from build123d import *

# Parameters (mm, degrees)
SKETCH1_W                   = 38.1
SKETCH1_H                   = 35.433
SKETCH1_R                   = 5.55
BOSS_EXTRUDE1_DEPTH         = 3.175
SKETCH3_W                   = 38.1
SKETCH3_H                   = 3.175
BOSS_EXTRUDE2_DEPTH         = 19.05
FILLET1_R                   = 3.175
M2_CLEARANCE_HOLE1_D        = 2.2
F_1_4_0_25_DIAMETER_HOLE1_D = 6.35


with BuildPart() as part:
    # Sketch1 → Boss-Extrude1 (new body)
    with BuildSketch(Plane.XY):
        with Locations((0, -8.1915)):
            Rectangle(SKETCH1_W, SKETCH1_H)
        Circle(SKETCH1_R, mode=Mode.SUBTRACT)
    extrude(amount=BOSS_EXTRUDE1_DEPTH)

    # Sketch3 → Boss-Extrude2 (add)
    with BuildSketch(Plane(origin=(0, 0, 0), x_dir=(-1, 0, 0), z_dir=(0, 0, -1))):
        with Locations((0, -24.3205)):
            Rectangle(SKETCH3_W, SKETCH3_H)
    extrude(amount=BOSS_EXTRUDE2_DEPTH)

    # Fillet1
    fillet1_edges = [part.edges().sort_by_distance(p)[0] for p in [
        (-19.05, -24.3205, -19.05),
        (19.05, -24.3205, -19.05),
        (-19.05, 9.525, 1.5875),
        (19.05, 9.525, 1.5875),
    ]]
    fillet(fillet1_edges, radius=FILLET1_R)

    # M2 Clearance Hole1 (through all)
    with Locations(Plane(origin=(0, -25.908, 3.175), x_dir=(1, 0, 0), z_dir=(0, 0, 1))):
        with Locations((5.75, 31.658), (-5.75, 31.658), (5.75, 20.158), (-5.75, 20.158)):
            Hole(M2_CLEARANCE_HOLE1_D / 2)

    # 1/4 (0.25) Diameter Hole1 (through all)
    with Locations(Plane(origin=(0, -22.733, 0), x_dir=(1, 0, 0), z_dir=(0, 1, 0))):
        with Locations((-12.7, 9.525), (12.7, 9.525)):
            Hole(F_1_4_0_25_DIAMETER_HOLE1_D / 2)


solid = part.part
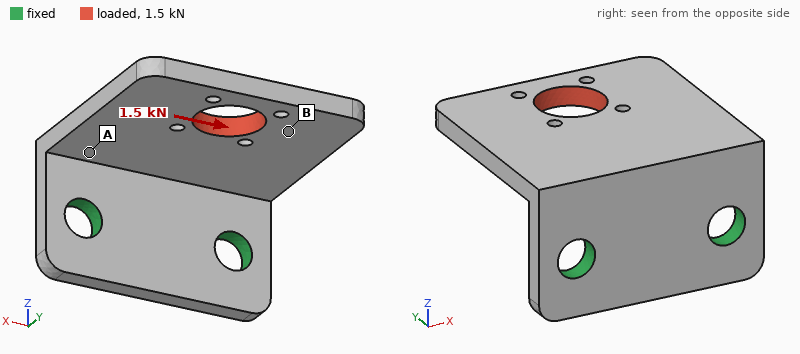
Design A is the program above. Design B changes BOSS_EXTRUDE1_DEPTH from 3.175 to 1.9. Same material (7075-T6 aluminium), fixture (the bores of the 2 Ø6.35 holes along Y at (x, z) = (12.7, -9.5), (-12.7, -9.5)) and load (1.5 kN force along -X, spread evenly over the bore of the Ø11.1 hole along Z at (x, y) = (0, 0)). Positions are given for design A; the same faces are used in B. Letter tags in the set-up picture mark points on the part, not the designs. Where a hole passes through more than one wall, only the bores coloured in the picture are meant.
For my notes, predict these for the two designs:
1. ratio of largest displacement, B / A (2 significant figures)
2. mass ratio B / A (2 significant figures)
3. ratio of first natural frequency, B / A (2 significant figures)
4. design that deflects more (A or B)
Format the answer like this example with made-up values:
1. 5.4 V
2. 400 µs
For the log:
1. 1.2
2. 0.74
3. 0.80
4. B
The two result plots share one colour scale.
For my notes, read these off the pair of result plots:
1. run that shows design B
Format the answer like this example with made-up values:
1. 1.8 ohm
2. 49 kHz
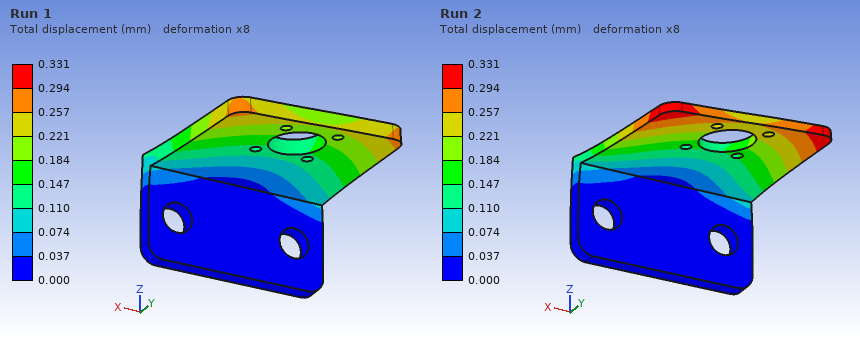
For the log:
1. Run 2
